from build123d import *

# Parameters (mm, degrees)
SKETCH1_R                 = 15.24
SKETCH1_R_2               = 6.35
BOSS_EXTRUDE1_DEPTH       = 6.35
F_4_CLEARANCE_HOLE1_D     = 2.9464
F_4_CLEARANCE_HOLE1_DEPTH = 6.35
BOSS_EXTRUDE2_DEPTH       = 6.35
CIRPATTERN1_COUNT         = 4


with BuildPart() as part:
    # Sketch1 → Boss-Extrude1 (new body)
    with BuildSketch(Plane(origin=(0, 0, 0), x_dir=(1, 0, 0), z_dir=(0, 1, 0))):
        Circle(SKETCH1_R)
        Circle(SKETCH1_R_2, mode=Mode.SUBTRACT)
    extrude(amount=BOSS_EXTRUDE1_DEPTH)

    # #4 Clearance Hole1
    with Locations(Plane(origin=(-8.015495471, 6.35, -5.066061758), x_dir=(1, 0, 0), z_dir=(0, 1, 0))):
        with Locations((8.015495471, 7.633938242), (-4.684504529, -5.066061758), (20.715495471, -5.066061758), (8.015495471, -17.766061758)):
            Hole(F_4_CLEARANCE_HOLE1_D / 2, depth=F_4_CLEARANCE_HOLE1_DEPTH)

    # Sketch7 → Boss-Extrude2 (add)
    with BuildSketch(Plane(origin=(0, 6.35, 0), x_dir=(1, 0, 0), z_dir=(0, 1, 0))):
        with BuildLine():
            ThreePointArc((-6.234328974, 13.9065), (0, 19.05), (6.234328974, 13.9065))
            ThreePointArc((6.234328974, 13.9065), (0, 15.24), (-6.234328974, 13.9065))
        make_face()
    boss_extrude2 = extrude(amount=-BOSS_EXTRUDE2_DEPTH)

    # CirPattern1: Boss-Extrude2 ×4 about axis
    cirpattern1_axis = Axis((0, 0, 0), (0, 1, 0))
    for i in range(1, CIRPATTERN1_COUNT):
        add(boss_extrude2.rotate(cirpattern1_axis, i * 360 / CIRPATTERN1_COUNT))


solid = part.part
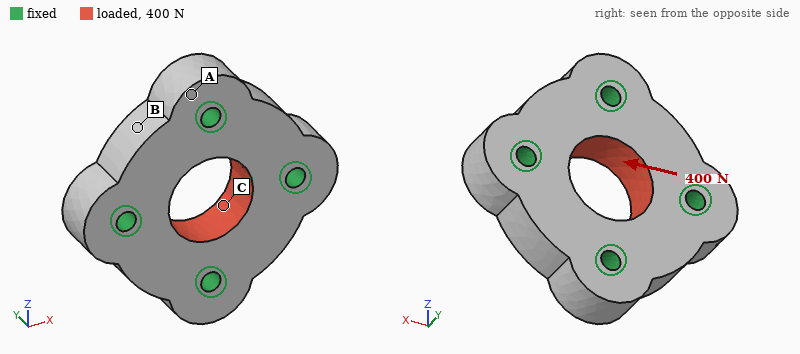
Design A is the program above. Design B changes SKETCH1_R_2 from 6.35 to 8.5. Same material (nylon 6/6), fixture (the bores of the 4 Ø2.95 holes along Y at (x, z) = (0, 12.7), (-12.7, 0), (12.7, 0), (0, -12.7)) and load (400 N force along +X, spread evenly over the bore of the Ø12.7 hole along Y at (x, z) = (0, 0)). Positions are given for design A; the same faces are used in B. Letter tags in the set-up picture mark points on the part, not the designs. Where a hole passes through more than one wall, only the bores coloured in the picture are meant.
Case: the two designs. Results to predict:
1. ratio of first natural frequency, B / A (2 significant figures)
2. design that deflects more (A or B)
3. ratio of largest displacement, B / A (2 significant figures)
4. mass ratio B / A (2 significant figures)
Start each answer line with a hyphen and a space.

- 1.0
- A
- 0.92
- 0.86
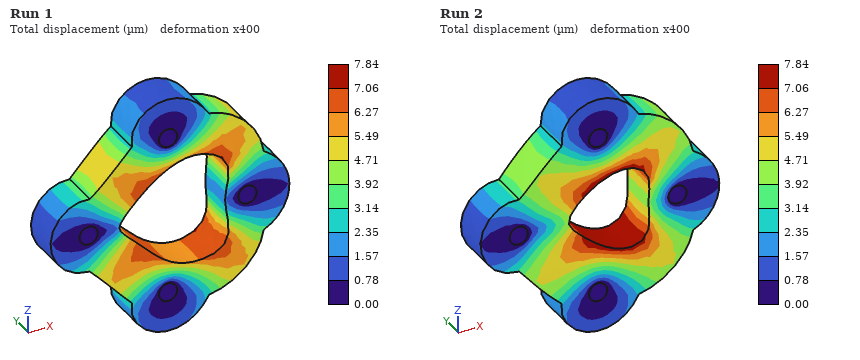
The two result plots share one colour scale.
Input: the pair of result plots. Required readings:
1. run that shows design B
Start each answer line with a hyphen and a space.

- Run 1
